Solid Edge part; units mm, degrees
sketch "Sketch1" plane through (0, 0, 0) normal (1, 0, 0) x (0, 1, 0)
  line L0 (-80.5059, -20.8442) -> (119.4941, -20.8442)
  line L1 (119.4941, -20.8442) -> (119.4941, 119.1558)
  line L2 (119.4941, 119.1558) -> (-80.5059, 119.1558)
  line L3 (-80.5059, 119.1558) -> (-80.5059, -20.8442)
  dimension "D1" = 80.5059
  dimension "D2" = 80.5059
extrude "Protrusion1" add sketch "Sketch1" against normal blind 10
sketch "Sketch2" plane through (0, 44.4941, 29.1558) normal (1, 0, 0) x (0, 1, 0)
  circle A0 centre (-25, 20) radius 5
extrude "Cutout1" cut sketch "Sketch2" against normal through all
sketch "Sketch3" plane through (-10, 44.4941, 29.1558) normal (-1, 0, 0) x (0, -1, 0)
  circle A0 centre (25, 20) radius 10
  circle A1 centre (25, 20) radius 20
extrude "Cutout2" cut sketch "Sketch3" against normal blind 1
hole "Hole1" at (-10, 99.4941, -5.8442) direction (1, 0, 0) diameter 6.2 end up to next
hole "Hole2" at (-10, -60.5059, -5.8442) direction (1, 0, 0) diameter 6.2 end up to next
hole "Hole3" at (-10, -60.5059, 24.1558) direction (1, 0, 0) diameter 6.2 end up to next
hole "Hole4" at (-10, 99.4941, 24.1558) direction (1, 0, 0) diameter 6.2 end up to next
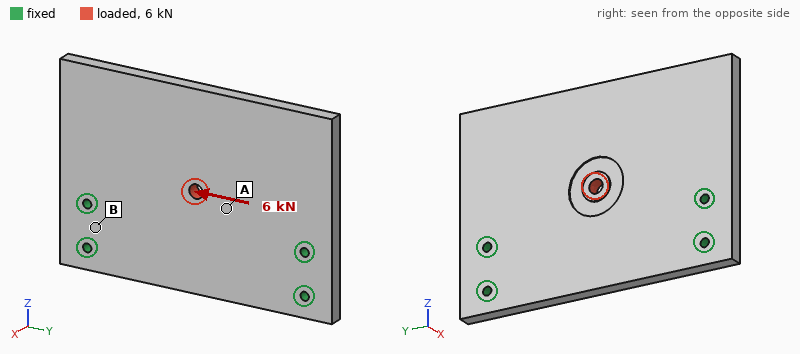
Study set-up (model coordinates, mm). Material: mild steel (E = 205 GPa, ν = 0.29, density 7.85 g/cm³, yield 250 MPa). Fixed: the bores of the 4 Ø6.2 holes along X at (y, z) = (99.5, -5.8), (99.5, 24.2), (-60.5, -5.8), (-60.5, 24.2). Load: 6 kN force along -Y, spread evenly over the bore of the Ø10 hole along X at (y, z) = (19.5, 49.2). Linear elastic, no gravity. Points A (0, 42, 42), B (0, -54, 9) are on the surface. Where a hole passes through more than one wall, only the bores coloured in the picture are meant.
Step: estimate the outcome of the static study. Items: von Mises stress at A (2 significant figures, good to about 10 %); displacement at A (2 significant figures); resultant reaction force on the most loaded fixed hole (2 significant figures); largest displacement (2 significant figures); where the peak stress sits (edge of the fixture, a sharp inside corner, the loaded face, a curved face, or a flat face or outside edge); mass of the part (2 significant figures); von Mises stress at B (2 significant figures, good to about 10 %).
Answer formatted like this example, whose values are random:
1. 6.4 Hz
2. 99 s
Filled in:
1. 9.2 MPa
2. 2.2 µm
3. 2.2 kN
4. 3.7 µm
5. the loaded face
6. 2.2 kg
7. 2.8 MPa
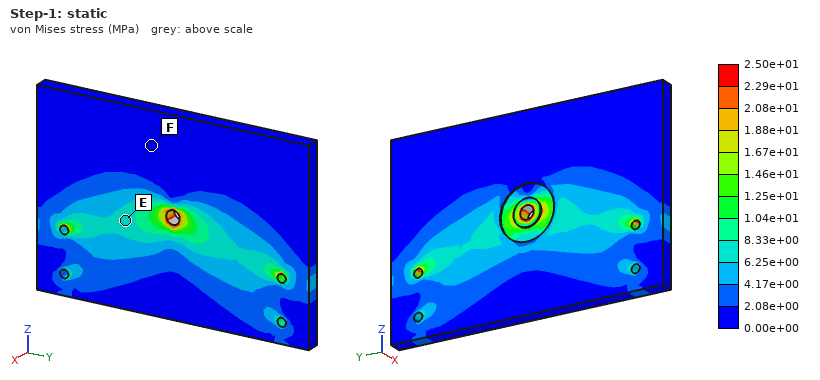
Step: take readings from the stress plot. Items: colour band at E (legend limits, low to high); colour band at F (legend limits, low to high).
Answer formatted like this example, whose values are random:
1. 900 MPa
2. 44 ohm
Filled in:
1. 6.25e+00 to 8.33e+00 MPa
2. 0.00e+00 to 2.08e+00 MPa
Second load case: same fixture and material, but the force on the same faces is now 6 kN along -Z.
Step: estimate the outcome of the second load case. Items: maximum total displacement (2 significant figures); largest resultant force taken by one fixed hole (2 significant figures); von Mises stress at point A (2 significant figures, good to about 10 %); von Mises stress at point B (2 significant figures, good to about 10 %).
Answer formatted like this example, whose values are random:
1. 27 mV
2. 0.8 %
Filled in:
1. 4.8 µm
2. 2.0 kN
3. 4.9 MPa
4. 6.1 MPa
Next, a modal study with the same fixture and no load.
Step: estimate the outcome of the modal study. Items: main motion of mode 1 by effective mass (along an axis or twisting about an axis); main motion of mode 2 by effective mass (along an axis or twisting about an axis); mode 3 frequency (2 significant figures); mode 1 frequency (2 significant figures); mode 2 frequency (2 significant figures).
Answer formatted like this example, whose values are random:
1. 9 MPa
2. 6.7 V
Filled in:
1. along X
2. twisting about Z
3. 1800 Hz
4. 680 Hz
5. 1300 Hz
